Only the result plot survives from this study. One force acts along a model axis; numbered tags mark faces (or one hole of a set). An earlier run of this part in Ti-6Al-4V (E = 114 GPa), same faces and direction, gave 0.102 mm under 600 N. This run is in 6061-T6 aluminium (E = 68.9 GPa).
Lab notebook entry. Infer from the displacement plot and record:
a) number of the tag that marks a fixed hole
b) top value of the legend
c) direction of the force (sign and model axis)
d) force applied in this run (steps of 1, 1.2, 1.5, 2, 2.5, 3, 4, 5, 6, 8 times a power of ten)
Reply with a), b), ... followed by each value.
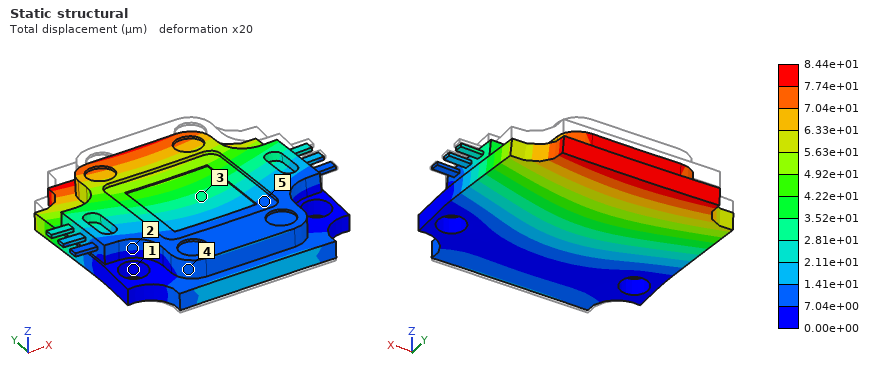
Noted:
a) 1
b) 8.44e+01 µm
c) -Z
d) 300 N
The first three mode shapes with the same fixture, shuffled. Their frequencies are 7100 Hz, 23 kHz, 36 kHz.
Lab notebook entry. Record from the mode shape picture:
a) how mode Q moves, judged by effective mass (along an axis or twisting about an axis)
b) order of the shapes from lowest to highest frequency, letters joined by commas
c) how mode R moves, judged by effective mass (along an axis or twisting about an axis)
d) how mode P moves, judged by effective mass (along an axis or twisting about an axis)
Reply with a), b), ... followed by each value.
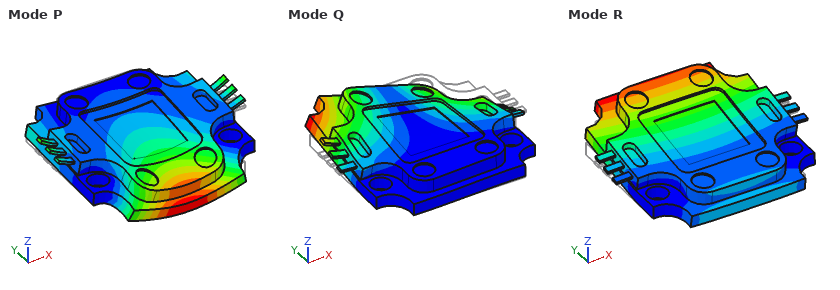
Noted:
a) twisting about Y
b) R, Q, P
c) along Z
d) along Z
